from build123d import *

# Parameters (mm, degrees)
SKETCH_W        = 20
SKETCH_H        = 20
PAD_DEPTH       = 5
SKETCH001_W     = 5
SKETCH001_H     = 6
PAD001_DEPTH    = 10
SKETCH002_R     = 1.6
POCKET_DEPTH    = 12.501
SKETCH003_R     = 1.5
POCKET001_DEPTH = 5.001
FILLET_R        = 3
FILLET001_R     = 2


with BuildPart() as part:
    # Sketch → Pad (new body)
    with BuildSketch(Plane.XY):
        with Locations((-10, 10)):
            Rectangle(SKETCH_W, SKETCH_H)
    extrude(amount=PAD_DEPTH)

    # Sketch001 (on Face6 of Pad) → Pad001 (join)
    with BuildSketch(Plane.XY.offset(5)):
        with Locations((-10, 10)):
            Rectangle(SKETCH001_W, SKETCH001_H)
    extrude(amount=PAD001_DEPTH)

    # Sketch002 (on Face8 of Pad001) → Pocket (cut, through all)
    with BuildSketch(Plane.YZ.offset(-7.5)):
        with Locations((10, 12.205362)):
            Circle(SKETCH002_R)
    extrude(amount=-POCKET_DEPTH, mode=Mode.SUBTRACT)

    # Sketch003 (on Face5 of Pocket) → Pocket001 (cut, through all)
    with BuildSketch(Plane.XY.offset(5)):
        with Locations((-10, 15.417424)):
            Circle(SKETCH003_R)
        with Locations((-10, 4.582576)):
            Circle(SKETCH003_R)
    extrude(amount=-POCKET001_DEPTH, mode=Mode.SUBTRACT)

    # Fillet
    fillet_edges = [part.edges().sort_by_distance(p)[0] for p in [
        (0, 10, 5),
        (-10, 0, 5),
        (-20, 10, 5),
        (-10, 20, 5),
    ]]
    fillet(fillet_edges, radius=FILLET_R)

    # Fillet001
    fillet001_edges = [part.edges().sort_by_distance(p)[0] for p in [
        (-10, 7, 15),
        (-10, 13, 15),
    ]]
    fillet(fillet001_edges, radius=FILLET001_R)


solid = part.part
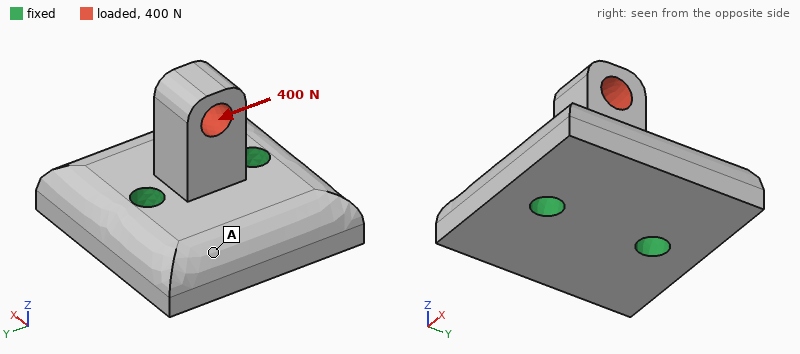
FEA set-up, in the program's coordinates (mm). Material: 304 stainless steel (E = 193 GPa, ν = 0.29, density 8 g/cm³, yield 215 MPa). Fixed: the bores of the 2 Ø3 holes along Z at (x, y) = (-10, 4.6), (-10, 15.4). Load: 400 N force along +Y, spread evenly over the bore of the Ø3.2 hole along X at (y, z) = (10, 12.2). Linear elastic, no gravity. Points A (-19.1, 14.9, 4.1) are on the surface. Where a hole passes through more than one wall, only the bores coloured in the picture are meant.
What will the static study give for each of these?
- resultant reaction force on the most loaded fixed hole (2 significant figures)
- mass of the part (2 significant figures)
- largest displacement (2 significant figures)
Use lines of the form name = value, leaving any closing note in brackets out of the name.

resultant reaction force on the most loaded fixed hole = 440 N
mass of the part = 16 g
largest displacement = 10 µm
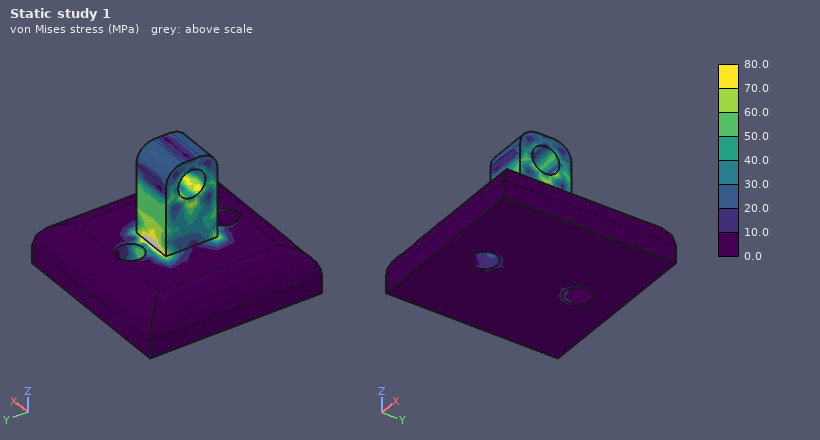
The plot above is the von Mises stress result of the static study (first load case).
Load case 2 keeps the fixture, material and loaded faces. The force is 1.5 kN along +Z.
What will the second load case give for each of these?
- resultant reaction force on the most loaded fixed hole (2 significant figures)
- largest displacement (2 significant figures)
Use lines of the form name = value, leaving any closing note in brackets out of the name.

resultant reaction force on the most loaded fixed hole = 760 N
largest displacement = 5.1 µm
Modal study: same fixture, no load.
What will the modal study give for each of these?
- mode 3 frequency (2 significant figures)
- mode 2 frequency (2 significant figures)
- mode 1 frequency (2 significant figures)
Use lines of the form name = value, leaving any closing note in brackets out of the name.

mode 3 frequency = 40 kHz
mode 2 frequency = 36 kHz
mode 1 frequency = 28 kHz
